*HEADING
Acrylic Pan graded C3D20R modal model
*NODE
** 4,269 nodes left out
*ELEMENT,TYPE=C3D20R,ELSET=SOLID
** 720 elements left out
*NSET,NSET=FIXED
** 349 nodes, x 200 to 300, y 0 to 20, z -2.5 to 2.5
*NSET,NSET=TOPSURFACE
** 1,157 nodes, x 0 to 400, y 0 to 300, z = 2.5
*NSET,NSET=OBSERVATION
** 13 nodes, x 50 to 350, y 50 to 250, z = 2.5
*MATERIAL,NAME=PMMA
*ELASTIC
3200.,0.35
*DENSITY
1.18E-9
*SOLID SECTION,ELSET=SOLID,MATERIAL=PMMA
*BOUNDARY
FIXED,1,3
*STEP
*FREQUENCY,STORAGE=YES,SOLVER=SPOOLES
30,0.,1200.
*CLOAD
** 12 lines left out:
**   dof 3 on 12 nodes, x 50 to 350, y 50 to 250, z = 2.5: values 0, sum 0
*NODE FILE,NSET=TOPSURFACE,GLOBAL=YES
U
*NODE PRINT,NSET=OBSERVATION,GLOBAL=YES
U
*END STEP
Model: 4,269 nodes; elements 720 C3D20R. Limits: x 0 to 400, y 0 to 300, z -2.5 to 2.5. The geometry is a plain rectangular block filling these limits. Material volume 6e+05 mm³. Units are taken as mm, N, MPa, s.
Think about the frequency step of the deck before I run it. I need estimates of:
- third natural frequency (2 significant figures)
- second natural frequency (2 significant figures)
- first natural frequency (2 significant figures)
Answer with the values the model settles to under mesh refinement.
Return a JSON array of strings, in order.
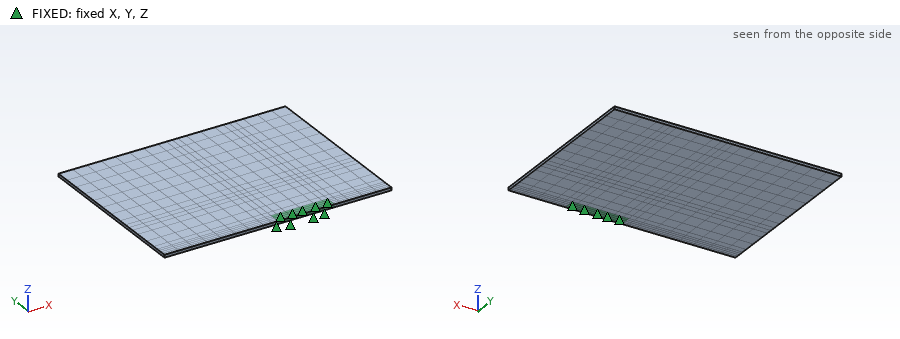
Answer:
["44 Hz", "21 Hz", "13 Hz"]
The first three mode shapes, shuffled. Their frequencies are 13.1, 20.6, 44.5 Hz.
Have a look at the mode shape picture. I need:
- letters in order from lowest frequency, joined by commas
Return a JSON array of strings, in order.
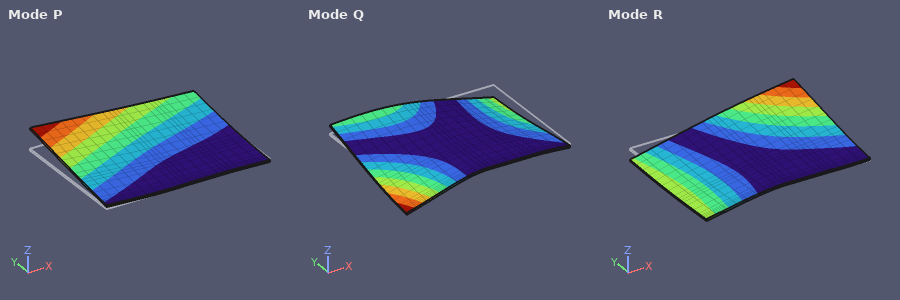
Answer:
["P, R, Q"]
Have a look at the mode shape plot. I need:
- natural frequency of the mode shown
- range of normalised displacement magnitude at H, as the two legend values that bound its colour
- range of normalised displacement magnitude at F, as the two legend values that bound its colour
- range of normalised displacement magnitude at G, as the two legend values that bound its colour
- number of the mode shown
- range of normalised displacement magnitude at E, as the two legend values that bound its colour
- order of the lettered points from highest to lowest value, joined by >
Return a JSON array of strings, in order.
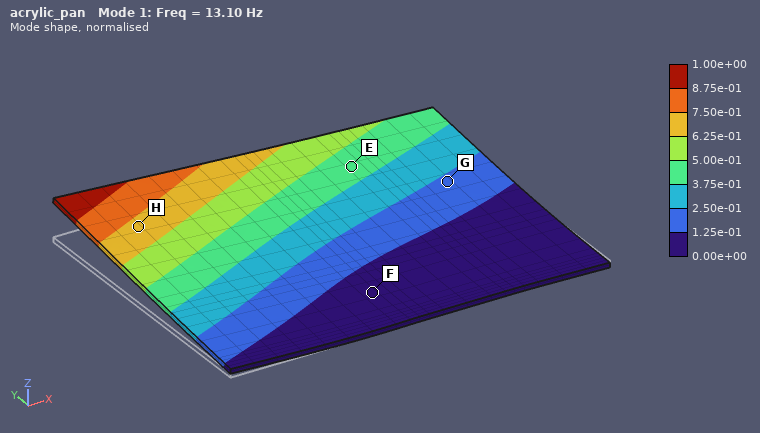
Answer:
["13.10 Hz", "6.25e-01 to 7.50e-01", "0.00e+00 to 1.25e-01", "1.25e-01 to 2.50e-01", "1", "3.75e-01 to 5.00e-01", "H > E > G > F"]
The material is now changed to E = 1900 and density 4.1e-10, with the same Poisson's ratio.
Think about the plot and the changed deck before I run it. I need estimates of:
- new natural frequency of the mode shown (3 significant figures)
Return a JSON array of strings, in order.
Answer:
["17.1 Hz"]
